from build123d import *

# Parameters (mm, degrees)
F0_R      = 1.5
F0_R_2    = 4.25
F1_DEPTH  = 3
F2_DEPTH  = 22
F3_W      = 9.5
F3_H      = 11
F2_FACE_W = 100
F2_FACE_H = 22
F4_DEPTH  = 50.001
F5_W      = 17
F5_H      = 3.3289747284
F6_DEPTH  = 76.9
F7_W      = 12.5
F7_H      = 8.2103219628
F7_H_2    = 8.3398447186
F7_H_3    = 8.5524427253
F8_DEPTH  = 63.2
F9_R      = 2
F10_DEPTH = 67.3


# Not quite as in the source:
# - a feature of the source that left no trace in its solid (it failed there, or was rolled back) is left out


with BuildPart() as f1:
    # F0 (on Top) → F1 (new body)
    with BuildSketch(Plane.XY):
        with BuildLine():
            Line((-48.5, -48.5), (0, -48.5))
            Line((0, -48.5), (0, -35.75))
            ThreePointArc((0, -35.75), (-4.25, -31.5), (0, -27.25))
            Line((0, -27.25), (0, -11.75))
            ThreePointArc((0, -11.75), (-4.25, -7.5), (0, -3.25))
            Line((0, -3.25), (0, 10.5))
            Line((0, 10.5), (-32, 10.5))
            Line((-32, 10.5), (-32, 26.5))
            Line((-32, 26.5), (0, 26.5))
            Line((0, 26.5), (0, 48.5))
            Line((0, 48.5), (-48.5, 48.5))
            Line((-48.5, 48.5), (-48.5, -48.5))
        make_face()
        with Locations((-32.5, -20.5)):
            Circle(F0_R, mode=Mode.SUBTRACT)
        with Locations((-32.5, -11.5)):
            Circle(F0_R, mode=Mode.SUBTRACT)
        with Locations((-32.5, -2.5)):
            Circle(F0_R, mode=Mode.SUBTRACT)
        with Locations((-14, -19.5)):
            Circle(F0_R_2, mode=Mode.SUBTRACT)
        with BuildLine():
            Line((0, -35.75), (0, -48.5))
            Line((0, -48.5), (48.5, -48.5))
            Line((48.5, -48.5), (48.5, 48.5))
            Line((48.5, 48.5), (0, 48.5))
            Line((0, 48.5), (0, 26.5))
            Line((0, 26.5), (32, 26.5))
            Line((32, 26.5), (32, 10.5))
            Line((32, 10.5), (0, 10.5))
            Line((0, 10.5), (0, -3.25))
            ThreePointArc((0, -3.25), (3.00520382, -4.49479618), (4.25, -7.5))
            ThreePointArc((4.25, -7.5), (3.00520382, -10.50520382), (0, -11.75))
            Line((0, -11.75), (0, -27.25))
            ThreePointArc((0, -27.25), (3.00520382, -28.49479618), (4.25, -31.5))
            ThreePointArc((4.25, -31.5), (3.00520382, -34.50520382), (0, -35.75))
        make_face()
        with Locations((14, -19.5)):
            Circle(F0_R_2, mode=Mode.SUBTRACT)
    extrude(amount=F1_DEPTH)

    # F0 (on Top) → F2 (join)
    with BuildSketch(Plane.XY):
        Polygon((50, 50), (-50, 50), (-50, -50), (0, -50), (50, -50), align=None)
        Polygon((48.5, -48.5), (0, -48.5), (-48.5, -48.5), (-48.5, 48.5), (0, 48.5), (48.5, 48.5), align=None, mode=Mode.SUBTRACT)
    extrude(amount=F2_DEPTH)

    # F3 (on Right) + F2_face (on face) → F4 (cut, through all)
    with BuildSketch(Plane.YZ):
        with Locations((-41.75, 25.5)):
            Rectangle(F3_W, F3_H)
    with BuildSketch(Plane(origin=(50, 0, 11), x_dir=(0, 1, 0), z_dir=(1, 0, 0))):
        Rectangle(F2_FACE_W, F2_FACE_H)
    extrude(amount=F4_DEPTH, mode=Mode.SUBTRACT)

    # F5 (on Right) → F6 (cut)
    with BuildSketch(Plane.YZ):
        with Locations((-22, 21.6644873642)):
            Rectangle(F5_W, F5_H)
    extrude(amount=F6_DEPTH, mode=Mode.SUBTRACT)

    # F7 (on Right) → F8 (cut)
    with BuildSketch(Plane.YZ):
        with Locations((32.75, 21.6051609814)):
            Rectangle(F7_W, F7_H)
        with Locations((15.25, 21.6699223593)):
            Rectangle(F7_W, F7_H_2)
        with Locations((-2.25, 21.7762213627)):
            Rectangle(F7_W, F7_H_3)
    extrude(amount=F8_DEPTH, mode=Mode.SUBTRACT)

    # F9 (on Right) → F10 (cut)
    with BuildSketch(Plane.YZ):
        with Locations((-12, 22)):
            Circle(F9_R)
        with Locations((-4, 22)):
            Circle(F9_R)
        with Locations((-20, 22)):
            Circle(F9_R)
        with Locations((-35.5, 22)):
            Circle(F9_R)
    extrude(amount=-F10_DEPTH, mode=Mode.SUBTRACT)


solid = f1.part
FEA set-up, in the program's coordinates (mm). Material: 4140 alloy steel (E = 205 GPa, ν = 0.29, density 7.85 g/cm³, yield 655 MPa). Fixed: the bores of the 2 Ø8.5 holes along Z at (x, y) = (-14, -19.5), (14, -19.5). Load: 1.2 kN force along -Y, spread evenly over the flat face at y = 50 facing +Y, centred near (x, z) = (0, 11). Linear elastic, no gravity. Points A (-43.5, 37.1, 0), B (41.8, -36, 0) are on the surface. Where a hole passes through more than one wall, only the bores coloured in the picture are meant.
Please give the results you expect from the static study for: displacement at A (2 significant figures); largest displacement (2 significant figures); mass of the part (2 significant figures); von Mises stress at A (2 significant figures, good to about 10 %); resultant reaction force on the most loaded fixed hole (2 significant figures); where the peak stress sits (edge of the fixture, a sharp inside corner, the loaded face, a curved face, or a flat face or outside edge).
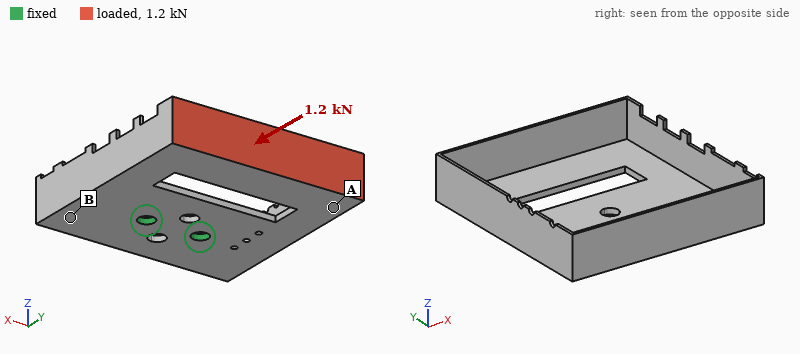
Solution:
0.22 mm
0.44 mm
290 g
48 MPa
600 N
the loaded face
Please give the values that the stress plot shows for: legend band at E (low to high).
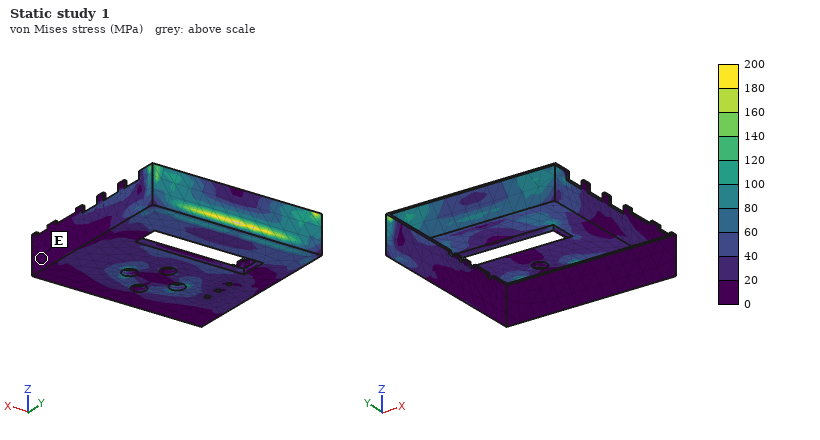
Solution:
0 to 20 MPa
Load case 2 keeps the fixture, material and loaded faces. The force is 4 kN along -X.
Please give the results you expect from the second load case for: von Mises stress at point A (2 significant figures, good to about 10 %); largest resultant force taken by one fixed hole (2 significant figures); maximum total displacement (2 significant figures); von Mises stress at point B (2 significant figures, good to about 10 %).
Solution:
140 MPa
7.5 kN
1.5 mm
180 MPa
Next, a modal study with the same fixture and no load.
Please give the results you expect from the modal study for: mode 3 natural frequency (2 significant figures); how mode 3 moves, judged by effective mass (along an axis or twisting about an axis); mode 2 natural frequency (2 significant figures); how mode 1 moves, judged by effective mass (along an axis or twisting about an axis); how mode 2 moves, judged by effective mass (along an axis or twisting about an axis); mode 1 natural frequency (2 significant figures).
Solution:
1300 Hz
twisting about Y
610 Hz
along Z
twisting about Y
440 Hz
